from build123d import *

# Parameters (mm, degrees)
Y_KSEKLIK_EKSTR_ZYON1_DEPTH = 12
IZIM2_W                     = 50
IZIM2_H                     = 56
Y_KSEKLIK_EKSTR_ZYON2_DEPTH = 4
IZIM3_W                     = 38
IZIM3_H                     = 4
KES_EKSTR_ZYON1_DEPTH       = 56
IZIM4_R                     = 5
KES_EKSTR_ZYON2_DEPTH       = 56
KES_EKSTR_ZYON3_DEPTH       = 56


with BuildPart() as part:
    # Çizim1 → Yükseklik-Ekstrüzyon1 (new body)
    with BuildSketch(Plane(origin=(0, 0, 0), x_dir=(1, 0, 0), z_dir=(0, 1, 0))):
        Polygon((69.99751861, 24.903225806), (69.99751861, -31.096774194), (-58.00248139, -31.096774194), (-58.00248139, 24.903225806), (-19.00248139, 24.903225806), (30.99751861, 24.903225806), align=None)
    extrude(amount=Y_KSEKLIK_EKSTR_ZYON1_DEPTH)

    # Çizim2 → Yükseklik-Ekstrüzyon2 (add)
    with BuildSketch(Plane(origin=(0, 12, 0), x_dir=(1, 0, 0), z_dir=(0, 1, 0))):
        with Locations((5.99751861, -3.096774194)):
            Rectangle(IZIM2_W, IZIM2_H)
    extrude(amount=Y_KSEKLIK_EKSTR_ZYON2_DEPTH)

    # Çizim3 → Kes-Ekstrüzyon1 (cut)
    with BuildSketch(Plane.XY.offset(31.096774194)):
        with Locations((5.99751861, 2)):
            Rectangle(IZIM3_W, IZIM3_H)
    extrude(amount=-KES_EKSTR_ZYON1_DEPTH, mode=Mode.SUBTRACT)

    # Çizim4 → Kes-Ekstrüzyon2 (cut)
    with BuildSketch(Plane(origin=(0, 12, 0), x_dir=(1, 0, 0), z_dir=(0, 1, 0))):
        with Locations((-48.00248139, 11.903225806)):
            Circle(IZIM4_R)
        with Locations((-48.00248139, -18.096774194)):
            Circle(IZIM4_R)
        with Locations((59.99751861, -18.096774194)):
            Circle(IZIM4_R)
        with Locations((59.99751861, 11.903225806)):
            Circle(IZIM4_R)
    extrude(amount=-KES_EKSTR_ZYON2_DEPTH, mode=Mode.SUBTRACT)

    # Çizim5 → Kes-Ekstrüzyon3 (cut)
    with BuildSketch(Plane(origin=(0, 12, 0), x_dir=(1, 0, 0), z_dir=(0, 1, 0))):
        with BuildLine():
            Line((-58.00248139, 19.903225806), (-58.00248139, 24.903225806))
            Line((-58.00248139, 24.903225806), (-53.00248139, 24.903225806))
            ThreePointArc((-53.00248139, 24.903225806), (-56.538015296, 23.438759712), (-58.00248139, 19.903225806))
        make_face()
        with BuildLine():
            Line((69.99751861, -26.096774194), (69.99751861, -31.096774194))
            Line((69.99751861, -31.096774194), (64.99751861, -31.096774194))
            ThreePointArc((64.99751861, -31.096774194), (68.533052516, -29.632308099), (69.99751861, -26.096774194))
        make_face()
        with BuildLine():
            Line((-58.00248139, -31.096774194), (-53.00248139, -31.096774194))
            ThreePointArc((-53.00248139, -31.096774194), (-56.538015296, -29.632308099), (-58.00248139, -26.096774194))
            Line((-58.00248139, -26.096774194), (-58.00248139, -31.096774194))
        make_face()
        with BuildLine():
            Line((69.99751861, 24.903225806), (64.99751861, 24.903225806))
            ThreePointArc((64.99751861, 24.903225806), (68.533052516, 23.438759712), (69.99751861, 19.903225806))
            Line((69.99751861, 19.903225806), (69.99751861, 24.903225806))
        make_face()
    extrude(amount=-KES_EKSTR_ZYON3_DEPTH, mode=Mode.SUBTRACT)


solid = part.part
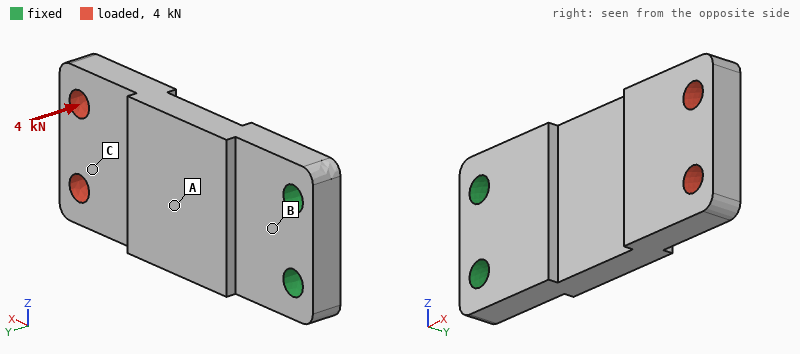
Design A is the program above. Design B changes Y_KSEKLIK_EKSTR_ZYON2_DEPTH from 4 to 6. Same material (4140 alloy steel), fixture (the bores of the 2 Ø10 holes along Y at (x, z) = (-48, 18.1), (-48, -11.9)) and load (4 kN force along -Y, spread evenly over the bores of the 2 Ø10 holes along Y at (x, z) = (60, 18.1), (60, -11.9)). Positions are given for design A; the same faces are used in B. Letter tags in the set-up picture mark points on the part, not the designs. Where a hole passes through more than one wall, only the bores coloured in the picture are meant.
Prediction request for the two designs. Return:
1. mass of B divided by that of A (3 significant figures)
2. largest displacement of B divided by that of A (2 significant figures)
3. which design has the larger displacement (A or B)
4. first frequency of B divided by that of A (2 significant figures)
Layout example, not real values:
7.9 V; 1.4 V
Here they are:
1.07; 0.89; A; 1.0
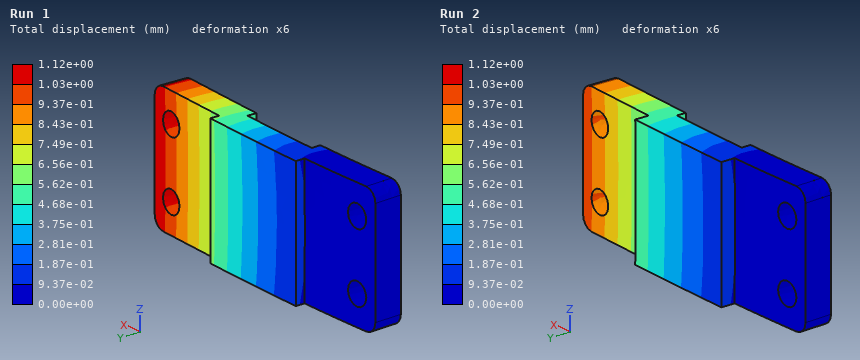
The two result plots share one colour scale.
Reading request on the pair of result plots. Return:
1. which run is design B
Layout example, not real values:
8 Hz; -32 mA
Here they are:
Run 2
